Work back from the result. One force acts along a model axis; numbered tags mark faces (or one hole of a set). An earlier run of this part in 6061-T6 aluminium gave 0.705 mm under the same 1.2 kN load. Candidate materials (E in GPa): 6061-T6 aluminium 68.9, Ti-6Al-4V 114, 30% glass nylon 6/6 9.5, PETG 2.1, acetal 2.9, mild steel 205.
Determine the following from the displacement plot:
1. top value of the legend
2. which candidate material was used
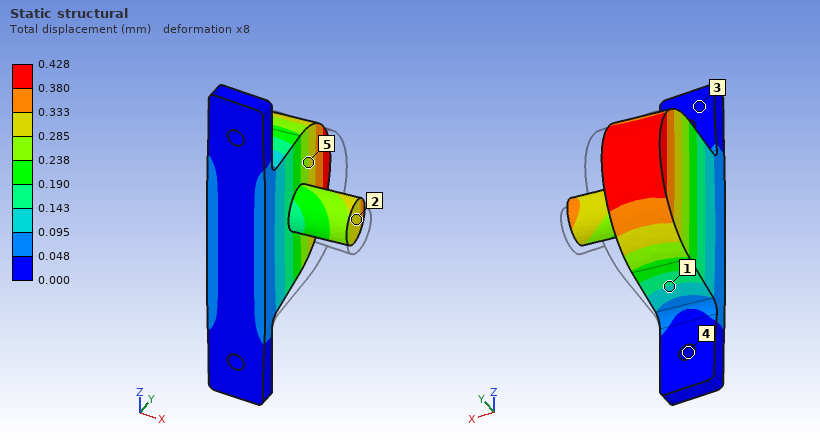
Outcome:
0.428 mm
Ti-6Al-4V
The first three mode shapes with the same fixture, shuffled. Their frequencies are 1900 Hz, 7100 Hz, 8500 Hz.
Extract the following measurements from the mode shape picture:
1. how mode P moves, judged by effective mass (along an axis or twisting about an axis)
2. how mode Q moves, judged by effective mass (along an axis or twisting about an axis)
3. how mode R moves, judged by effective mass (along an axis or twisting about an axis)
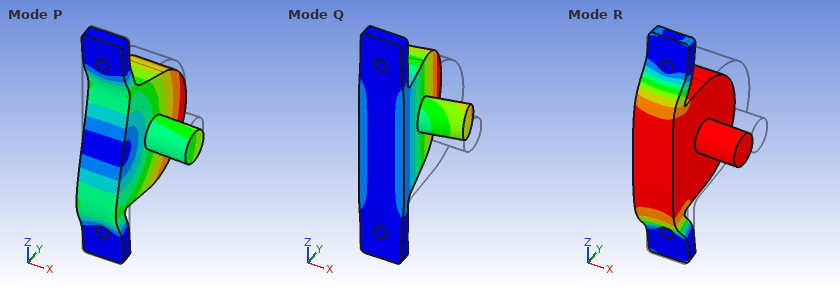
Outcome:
along Z
along X
along Y
